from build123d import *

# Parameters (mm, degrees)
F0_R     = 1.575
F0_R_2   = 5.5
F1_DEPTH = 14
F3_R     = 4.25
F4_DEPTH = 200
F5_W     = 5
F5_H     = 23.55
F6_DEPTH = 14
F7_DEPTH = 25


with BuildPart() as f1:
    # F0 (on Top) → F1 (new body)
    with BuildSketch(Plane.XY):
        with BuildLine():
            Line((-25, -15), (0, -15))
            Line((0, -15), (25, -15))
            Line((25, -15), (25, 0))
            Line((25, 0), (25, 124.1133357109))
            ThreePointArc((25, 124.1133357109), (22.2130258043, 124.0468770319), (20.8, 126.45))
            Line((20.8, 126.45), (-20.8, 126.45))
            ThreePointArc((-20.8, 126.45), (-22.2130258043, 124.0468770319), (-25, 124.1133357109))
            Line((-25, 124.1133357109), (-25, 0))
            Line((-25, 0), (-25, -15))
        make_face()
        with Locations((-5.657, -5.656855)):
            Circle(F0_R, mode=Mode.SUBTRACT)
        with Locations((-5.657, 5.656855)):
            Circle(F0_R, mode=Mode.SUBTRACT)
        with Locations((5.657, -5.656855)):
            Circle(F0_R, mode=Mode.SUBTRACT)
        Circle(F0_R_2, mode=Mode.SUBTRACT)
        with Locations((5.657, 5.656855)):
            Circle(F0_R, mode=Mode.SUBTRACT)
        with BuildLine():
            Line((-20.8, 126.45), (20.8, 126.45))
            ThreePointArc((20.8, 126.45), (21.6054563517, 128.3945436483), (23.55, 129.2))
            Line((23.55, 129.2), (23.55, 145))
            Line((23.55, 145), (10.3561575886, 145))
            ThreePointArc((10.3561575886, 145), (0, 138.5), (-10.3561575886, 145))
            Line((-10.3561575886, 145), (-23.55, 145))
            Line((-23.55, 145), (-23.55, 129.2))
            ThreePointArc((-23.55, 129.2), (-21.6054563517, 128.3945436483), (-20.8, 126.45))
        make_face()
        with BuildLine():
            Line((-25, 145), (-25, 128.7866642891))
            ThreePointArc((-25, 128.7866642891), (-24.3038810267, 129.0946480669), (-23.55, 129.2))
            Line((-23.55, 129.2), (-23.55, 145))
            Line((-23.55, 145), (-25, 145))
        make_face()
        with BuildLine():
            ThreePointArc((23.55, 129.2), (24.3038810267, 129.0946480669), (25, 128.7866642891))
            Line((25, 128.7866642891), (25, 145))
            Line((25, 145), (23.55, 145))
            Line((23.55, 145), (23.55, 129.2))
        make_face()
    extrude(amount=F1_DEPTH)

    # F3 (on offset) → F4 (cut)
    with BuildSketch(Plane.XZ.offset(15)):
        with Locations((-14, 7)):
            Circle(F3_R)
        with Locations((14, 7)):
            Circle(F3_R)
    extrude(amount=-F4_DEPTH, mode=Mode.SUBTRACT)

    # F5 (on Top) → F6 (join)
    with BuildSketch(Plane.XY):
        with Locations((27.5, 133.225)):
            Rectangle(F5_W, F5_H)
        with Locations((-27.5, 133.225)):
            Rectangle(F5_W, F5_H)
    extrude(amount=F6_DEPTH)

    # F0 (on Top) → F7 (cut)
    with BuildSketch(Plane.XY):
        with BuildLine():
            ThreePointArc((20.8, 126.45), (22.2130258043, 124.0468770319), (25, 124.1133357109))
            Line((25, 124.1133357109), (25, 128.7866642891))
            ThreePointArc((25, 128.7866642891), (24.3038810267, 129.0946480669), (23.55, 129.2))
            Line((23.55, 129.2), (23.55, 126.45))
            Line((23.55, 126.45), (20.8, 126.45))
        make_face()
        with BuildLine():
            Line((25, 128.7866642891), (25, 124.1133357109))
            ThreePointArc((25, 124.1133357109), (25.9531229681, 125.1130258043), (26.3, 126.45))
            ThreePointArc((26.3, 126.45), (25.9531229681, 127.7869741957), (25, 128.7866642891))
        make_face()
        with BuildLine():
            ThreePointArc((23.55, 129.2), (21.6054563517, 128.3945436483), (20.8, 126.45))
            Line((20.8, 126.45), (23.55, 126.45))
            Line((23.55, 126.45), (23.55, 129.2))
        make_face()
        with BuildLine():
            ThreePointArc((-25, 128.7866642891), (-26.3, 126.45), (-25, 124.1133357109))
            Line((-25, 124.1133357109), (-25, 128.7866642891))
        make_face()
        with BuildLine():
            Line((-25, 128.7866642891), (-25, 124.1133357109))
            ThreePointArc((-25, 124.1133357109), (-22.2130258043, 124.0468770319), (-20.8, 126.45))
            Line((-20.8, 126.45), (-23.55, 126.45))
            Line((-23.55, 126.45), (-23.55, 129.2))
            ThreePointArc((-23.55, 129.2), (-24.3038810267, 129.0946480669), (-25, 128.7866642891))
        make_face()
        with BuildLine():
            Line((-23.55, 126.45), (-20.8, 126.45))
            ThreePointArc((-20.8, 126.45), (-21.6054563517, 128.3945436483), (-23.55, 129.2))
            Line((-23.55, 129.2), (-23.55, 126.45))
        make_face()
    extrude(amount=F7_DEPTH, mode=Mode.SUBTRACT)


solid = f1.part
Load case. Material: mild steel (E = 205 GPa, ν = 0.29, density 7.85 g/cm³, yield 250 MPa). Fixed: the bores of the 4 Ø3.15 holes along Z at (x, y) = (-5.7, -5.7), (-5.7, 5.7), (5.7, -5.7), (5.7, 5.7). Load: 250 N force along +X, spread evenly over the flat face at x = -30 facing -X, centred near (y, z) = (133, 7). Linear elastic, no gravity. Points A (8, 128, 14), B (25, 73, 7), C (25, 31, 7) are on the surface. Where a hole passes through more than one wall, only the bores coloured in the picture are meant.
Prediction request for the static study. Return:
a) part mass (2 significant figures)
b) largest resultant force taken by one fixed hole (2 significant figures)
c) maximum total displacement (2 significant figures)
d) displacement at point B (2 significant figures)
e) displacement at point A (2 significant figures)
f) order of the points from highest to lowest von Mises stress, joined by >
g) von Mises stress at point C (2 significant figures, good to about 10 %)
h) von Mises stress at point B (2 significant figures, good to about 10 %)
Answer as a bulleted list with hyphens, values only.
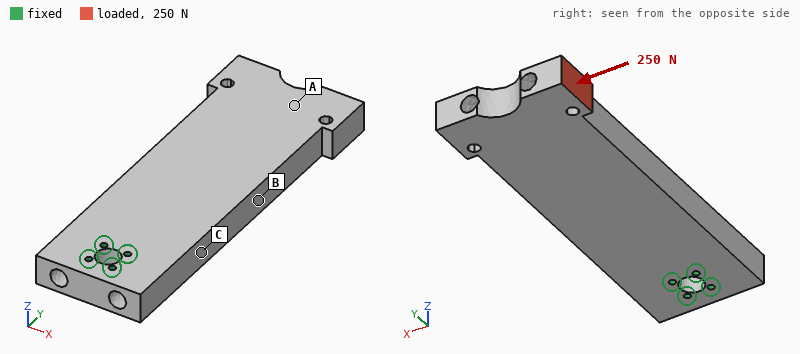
- 730 g
- 1.2 kN
- 16 µm
- 6.6 µm
- 13 µm
- C > B > A
- 5.3 MPa
- 3.0 MPa
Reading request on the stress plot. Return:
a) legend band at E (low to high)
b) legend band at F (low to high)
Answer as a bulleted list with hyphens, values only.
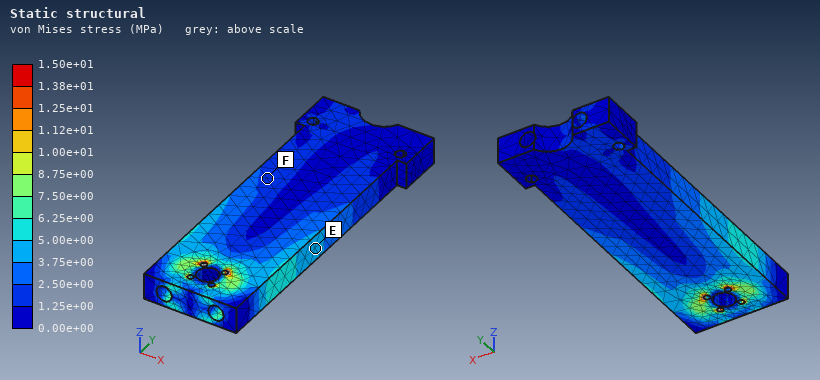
- 3.75e+00 to 5.00e+00 MPa
- 1.25e+00 to 2.50e+00 MPa
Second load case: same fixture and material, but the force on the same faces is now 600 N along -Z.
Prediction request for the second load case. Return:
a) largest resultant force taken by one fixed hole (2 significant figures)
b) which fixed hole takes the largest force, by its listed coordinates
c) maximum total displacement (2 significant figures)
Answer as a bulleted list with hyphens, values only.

- 1.3 kN
- (-5.7, 5.7)
- 0.26 mm
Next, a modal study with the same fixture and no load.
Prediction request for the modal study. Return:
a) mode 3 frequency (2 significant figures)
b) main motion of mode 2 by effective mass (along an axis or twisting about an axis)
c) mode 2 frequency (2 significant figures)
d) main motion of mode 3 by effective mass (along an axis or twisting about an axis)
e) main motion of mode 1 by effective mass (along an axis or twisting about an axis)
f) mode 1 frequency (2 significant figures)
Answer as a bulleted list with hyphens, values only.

- 2600 Hz
- along X
- 1400 Hz
- twisting about Y
- along Z
- 580 Hz
